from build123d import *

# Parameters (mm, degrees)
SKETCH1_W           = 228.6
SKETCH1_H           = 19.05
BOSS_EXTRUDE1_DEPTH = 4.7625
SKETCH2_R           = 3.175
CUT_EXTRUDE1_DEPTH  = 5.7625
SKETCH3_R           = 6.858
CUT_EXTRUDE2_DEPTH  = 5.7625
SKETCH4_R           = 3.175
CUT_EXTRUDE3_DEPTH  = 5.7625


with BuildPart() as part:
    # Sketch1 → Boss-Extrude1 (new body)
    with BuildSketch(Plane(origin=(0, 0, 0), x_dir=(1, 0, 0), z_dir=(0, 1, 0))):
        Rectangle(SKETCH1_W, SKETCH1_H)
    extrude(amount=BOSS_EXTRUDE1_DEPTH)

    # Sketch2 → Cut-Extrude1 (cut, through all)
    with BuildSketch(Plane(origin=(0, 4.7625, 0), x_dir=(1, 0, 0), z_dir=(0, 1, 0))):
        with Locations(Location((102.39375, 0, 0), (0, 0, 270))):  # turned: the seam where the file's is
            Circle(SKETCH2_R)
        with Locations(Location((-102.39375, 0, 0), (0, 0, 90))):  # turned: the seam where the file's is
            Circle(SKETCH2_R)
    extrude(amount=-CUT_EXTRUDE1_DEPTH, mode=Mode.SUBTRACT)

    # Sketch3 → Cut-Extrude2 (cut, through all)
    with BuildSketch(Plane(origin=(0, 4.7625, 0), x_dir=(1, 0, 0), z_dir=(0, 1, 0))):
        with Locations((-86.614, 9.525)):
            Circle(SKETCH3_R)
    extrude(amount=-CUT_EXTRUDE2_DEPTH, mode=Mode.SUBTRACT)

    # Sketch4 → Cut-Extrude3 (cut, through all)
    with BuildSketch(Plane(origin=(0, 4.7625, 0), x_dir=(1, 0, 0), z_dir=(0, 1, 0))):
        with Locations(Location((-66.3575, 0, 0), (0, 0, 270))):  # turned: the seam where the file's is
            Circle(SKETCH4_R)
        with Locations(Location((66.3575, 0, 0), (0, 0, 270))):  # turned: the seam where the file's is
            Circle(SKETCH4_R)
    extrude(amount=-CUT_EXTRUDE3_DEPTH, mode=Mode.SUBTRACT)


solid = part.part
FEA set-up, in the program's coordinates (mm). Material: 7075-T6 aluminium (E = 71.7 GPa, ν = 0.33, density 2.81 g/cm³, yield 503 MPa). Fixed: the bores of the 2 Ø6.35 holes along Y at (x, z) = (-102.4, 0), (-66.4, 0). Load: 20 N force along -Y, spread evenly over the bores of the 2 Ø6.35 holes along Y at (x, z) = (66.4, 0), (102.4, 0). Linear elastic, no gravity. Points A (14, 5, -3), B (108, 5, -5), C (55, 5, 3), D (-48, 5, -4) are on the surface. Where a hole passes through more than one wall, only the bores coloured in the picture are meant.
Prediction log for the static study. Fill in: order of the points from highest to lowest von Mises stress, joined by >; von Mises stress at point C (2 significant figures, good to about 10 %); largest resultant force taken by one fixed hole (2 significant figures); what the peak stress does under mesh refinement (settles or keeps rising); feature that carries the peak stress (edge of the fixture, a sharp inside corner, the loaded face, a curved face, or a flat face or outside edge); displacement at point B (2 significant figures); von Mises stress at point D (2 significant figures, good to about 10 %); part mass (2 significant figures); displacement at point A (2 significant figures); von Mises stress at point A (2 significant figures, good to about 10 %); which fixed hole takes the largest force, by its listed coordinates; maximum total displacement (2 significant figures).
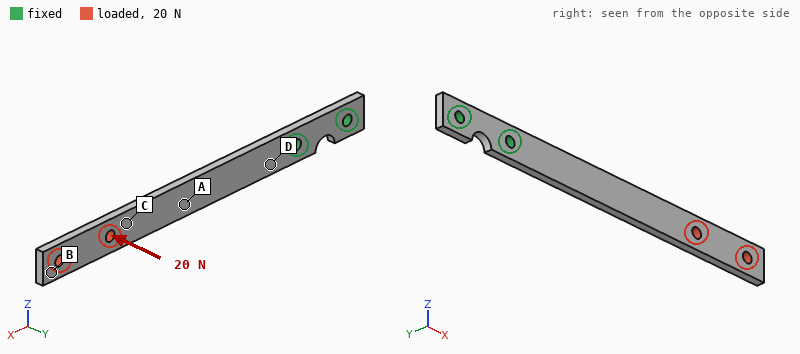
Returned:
D > A > C > B
8.3 MPa
21 N
keeps rising
edge of the fixture
2.2 mm
36 MPa
56 g
0.61 mm
20 MPa
(-66.4, 0)
2.3 mm
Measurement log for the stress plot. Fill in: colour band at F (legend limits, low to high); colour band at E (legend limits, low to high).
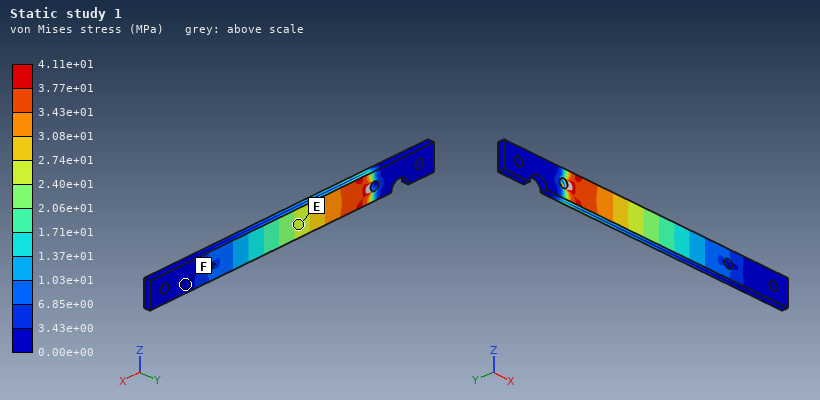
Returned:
0.00e+00 to 3.43e+00 MPa
2.40e+01 to 2.74e+01 MPa
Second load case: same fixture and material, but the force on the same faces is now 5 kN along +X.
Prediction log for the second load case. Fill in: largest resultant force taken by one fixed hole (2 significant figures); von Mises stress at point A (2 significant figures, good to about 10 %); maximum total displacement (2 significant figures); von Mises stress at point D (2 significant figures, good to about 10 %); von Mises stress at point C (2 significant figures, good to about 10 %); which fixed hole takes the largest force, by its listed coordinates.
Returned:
4.8 kN
55 MPa
0.12 mm
56 MPa
53 MPa
(-66.4, 0)
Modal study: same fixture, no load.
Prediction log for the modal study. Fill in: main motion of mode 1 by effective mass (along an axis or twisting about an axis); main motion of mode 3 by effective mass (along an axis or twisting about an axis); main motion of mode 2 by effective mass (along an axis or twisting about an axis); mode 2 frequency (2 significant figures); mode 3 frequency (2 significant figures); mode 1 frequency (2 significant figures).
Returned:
along Y
along Y
along Z
450 Hz
760 Hz
120 Hz
